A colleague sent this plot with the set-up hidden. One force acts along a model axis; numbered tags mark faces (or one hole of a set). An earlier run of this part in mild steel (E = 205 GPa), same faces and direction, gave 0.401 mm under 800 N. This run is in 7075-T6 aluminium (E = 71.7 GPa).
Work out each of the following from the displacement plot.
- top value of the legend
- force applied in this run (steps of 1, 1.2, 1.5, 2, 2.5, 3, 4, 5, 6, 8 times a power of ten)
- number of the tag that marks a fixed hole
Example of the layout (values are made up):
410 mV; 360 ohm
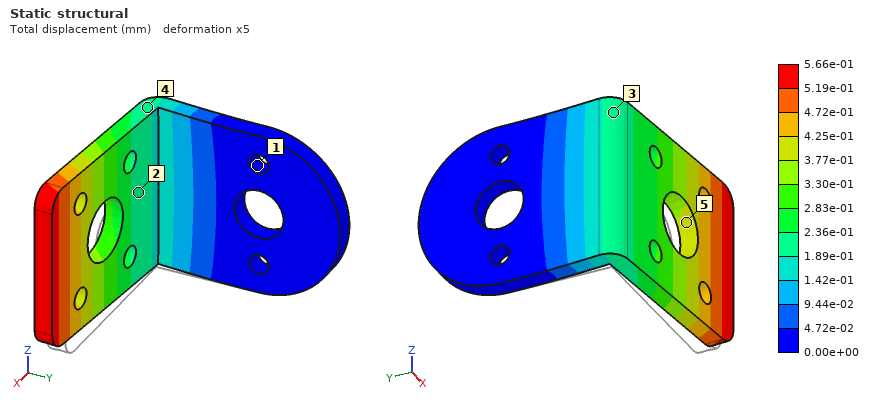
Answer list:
5.66e-01 mm; 400 N; 1
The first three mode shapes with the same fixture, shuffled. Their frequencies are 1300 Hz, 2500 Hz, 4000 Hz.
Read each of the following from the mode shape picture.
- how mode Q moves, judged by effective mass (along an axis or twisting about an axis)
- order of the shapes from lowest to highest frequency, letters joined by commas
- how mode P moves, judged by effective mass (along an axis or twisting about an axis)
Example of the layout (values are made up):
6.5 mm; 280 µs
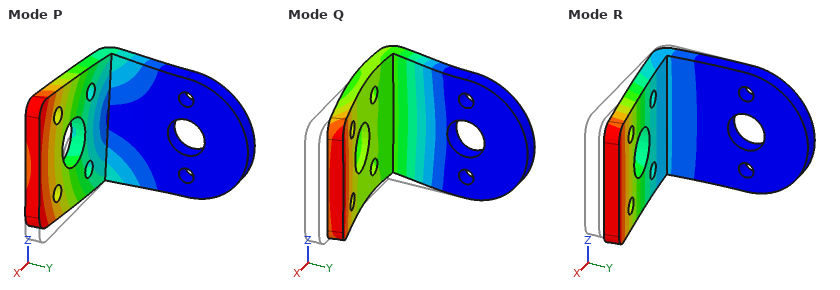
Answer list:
along X; R, P, Q; along Z
